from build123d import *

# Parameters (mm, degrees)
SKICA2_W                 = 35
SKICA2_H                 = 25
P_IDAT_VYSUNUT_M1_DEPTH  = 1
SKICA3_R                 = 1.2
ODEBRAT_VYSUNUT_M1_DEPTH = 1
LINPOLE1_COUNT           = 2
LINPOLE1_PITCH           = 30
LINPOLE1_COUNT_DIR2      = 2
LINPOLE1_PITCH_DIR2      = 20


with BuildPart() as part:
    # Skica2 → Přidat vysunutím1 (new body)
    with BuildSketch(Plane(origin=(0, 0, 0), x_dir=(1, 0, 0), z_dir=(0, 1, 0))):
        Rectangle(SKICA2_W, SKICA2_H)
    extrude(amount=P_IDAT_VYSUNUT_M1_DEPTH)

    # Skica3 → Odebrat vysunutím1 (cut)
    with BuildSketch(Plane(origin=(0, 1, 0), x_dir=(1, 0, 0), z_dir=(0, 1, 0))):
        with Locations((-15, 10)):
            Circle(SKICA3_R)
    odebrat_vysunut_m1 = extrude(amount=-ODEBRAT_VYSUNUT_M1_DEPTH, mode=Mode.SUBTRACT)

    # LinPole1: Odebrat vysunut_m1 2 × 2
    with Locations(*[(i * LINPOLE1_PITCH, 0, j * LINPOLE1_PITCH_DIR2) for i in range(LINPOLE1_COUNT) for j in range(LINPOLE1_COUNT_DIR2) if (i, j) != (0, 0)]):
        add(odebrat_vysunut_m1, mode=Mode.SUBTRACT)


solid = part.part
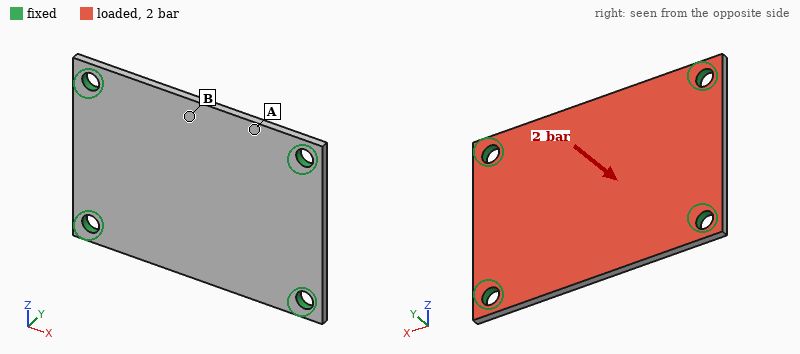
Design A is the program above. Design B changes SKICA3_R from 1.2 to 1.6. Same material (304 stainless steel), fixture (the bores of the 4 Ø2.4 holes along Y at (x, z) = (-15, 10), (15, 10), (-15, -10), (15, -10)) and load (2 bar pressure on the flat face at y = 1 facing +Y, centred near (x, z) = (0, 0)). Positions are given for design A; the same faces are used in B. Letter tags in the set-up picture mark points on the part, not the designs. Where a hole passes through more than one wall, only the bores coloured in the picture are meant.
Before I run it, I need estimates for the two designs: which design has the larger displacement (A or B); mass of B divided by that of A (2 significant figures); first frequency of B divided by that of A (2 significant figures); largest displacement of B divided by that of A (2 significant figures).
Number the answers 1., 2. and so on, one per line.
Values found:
1. A
2. 0.98
3. 1.1
4. 0.87
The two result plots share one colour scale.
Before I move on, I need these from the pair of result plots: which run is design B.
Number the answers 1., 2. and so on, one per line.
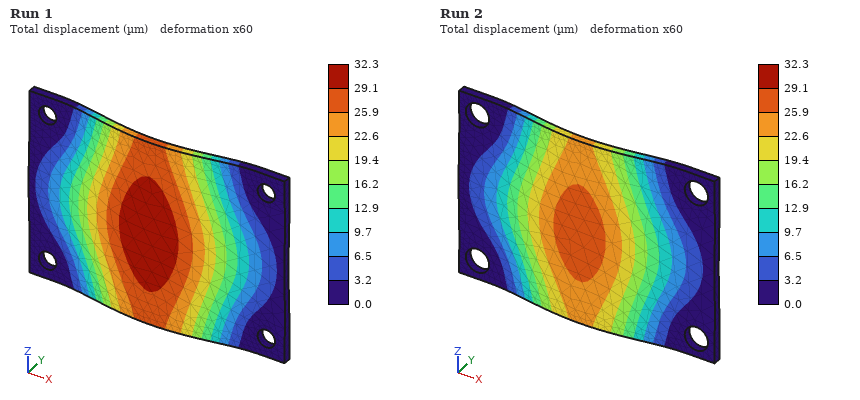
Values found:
1. Run 2
